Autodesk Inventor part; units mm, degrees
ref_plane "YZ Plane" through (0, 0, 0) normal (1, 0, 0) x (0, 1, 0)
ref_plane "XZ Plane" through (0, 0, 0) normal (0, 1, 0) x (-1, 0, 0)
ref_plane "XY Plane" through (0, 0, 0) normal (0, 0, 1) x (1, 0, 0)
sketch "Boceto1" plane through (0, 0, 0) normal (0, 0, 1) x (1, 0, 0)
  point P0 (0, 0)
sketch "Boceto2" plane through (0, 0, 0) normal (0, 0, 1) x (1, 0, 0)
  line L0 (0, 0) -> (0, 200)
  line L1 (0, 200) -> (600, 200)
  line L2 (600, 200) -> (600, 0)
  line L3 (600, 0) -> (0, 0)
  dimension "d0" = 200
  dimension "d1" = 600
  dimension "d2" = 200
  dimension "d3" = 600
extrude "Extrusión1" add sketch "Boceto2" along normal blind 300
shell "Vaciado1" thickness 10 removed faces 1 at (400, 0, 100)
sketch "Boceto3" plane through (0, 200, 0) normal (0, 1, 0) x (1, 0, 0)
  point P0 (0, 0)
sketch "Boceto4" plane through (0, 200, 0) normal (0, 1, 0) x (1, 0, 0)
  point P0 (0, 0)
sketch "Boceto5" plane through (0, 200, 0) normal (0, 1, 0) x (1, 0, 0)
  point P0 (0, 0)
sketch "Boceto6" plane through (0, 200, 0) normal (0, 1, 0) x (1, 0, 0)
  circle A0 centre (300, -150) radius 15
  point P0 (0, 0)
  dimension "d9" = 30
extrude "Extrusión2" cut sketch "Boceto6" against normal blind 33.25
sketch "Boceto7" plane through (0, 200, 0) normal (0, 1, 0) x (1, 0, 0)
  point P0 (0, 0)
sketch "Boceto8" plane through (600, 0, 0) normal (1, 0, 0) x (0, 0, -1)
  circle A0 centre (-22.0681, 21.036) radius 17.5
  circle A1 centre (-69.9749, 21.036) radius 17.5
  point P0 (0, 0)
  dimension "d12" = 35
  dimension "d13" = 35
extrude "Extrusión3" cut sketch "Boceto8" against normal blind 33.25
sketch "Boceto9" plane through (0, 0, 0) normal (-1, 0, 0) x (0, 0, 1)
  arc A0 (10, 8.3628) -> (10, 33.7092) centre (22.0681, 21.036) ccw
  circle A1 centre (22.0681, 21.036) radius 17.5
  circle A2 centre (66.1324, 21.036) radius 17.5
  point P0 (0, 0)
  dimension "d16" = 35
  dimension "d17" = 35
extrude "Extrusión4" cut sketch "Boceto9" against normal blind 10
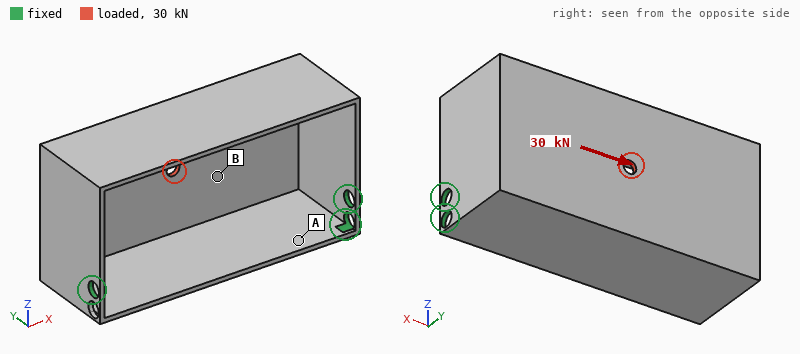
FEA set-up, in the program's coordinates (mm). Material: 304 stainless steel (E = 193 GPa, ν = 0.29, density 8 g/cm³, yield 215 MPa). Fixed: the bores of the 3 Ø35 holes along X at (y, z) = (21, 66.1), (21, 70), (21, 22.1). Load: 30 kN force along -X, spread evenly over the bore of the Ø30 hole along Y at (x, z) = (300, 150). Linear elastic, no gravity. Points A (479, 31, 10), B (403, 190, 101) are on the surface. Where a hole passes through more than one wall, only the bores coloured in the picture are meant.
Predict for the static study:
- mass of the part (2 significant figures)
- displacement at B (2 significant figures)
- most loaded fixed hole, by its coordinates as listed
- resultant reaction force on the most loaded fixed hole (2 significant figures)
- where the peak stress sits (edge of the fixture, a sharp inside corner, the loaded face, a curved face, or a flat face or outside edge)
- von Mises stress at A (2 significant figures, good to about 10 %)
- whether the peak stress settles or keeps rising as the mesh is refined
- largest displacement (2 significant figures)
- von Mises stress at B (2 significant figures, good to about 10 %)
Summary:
41 kg
0.11 mm
(21, 22.1)
34 kN
a sharp inside corner
26 MPa
keeps rising
0.36 mm
13 MPa
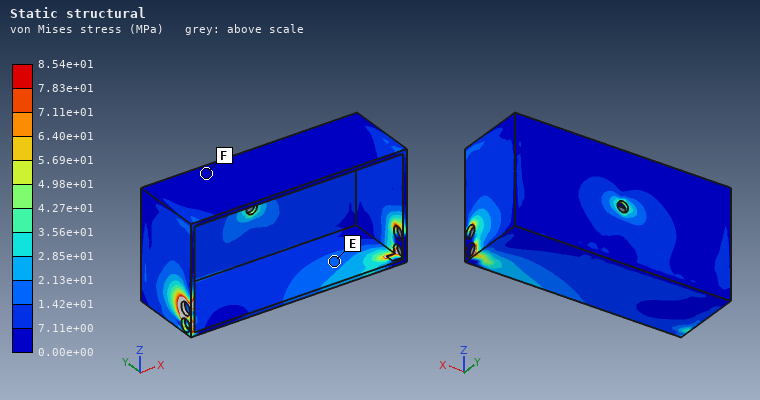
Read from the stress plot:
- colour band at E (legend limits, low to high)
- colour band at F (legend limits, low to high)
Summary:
1.42e+01 to 2.13e+01 MPa
0.00e+00 to 7.11e+00 MPa
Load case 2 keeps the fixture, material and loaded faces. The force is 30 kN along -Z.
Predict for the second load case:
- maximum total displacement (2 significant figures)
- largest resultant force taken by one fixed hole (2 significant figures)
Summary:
0.45 mm
33 kN
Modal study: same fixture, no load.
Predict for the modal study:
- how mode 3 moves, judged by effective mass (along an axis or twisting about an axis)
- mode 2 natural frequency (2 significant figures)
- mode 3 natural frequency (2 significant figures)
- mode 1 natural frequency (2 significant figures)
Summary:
along Z
230 Hz
260 Hz
220 Hz
